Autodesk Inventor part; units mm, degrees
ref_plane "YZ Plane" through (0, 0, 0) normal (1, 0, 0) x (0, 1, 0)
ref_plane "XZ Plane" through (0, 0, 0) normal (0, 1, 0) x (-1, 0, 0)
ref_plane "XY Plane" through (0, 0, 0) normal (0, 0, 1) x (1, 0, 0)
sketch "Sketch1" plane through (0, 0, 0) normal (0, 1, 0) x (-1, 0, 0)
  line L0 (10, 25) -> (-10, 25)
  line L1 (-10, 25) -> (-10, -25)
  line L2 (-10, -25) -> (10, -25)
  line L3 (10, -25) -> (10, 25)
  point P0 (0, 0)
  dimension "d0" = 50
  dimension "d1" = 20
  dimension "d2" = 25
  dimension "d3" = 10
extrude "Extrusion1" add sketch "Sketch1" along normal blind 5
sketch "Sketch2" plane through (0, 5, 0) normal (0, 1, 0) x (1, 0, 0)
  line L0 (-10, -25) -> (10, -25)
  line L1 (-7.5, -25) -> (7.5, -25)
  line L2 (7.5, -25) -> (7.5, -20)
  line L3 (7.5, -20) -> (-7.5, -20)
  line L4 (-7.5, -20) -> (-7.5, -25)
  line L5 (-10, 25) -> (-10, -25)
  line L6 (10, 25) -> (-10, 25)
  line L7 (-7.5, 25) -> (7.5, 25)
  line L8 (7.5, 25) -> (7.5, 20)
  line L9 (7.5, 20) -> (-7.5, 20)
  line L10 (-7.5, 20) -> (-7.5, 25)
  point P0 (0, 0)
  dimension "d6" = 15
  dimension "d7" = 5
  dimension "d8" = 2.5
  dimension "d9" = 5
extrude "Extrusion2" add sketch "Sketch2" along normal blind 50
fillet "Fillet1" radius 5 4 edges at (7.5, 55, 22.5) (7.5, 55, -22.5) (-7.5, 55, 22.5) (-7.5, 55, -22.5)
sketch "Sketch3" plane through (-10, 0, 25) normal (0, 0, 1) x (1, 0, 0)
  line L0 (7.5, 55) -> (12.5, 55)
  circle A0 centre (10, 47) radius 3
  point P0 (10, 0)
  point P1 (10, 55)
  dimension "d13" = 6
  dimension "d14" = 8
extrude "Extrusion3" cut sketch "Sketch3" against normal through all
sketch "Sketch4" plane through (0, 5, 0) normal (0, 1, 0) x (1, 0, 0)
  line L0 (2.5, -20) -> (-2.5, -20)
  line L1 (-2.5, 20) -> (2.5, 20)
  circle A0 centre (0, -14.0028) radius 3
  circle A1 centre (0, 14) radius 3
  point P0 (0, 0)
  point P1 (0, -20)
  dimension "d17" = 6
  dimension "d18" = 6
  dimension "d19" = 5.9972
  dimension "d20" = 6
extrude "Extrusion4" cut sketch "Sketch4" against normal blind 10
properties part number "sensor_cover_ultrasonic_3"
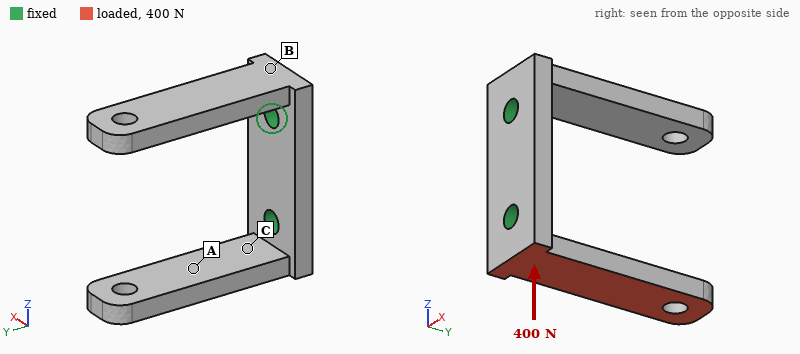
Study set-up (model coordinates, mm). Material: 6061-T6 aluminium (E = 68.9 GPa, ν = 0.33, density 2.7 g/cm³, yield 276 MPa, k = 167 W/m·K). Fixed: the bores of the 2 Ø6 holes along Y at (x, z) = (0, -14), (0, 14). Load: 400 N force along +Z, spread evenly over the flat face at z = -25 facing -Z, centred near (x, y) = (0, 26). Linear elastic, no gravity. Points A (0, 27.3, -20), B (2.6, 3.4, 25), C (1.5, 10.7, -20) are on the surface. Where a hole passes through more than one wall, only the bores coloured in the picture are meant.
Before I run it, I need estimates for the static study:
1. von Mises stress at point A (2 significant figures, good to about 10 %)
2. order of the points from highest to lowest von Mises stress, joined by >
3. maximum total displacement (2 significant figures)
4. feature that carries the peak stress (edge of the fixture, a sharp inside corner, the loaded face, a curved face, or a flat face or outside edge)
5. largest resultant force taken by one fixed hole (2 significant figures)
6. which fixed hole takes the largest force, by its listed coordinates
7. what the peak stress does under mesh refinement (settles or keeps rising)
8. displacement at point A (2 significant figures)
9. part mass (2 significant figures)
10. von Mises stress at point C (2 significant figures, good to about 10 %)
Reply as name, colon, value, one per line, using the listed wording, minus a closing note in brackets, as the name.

von Mises stress at point A: 39 MPa
order of the points from highest to lowest von Mises stress, joined by >: C > A > B
maximum total displacement: 0.76 mm
feature that carries the peak stress: edge of the fixture
largest resultant force taken by one fixed hole: 390 N
which fixed hole takes the largest force, by its listed coordinates: (0, -14)
what the peak stress does under mesh refinement: keeps rising
displacement at point A: 0.27 mm
part mass: 32 g
von Mises stress at point C: 99 MPa
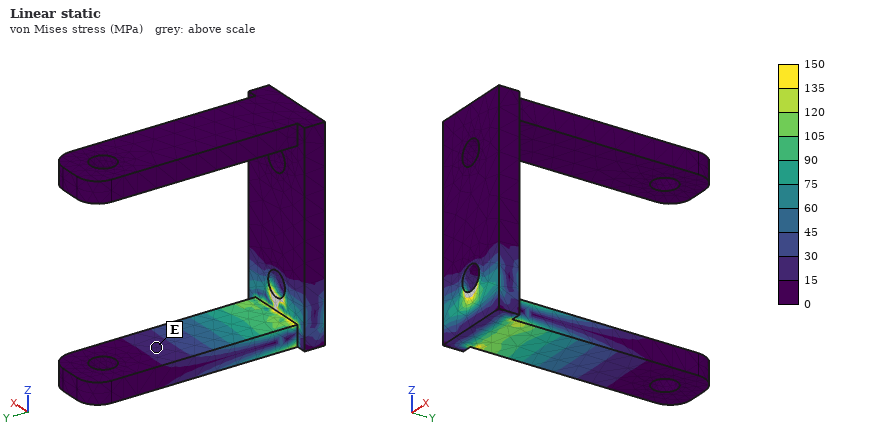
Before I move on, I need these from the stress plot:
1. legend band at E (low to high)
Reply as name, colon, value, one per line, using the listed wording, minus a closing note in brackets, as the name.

legend band at E: 15 to 30 MPa
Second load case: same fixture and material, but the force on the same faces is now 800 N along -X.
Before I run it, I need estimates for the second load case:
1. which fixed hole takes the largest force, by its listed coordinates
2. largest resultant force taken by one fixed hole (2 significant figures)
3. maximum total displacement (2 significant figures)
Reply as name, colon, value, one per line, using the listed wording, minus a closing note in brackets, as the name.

which fixed hole takes the largest force, by its listed coordinates: (0, -14)
largest resultant force taken by one fixed hole: 950 N
maximum total displacement: 0.38 mm
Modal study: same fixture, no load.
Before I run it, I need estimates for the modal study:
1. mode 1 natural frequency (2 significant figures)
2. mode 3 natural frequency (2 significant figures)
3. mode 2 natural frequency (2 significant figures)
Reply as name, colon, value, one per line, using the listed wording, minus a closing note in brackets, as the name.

mode 1 natural frequency: 1400 Hz
mode 3 natural frequency: 2700 Hz
mode 2 natural frequency: 1400 Hz
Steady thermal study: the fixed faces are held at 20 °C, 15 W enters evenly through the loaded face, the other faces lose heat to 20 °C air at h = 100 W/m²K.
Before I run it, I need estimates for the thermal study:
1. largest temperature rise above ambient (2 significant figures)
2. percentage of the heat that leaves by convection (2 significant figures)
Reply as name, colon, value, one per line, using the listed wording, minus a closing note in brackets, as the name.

largest temperature rise above ambient: 25 K
percentage of the heat that leaves by convection: 19 %
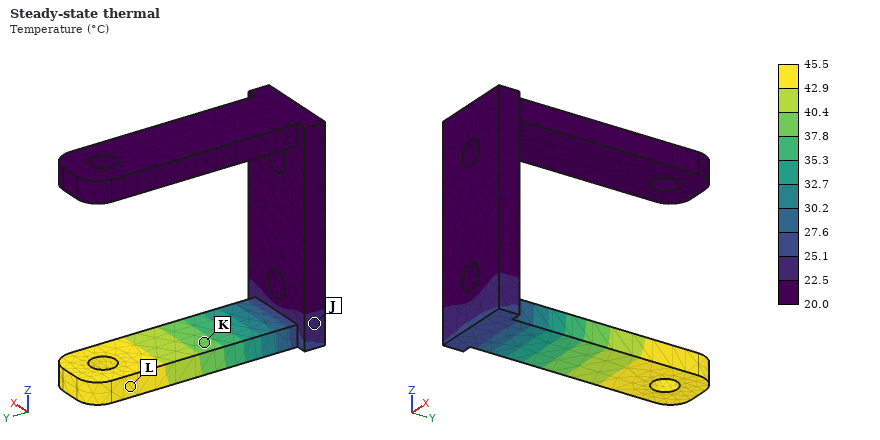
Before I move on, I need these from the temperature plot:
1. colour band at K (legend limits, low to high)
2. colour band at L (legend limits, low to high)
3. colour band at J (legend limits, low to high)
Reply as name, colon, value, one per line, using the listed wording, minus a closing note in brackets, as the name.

colour band at K: 37.8 to 40.4 °C
colour band at L: 42.9 to 45.5 °C
colour band at J: 22.5 to 25.1 °C
